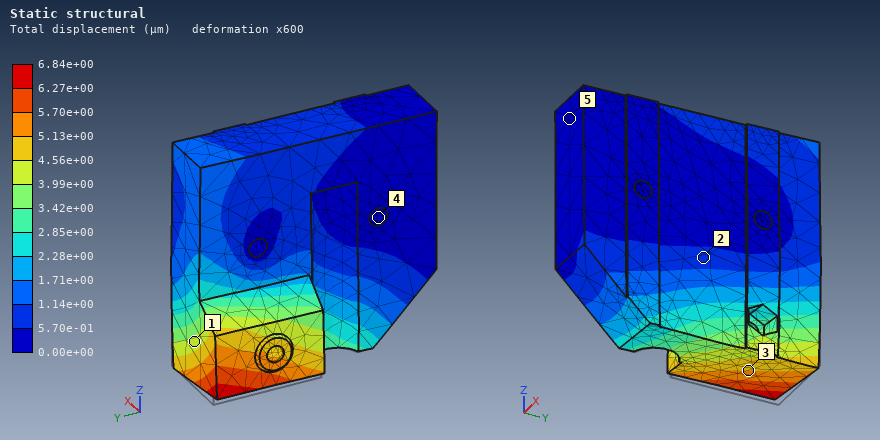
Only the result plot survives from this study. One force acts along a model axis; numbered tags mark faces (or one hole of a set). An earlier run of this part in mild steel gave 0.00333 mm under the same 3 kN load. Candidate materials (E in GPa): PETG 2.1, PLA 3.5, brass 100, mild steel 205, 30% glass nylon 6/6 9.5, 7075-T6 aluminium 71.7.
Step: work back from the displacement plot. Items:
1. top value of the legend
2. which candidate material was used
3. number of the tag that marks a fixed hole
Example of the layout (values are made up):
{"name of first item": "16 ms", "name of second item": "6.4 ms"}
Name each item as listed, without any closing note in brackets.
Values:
{"top value of the legend": "6.84e+00 µm", "which candidate material was used": "brass", "number of the tag that marks a fixed hole": "4"}
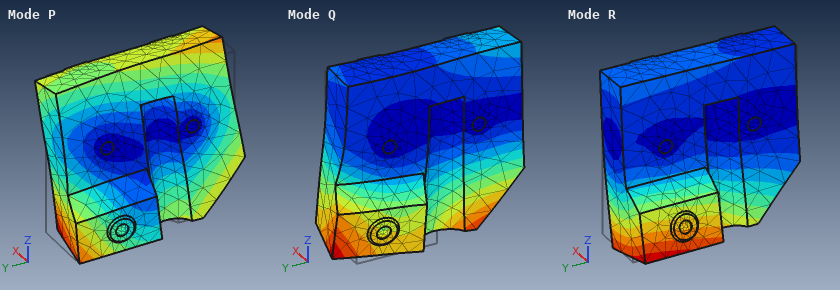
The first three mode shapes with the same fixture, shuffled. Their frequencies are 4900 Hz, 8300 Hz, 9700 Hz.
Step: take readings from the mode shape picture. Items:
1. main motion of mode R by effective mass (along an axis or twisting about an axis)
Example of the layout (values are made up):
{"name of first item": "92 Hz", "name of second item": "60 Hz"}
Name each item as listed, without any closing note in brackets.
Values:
{"main motion of mode R by effective mass": "along X"}
